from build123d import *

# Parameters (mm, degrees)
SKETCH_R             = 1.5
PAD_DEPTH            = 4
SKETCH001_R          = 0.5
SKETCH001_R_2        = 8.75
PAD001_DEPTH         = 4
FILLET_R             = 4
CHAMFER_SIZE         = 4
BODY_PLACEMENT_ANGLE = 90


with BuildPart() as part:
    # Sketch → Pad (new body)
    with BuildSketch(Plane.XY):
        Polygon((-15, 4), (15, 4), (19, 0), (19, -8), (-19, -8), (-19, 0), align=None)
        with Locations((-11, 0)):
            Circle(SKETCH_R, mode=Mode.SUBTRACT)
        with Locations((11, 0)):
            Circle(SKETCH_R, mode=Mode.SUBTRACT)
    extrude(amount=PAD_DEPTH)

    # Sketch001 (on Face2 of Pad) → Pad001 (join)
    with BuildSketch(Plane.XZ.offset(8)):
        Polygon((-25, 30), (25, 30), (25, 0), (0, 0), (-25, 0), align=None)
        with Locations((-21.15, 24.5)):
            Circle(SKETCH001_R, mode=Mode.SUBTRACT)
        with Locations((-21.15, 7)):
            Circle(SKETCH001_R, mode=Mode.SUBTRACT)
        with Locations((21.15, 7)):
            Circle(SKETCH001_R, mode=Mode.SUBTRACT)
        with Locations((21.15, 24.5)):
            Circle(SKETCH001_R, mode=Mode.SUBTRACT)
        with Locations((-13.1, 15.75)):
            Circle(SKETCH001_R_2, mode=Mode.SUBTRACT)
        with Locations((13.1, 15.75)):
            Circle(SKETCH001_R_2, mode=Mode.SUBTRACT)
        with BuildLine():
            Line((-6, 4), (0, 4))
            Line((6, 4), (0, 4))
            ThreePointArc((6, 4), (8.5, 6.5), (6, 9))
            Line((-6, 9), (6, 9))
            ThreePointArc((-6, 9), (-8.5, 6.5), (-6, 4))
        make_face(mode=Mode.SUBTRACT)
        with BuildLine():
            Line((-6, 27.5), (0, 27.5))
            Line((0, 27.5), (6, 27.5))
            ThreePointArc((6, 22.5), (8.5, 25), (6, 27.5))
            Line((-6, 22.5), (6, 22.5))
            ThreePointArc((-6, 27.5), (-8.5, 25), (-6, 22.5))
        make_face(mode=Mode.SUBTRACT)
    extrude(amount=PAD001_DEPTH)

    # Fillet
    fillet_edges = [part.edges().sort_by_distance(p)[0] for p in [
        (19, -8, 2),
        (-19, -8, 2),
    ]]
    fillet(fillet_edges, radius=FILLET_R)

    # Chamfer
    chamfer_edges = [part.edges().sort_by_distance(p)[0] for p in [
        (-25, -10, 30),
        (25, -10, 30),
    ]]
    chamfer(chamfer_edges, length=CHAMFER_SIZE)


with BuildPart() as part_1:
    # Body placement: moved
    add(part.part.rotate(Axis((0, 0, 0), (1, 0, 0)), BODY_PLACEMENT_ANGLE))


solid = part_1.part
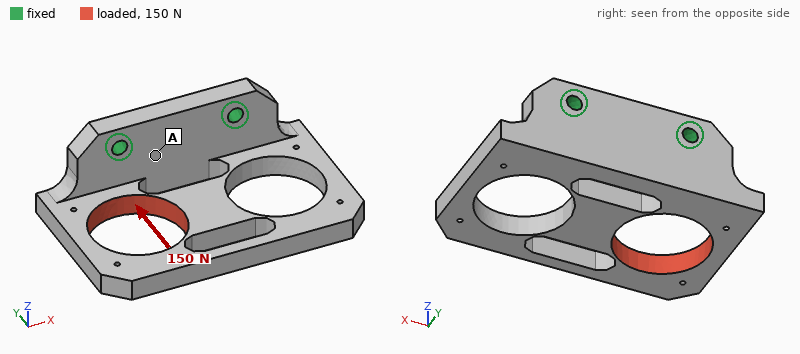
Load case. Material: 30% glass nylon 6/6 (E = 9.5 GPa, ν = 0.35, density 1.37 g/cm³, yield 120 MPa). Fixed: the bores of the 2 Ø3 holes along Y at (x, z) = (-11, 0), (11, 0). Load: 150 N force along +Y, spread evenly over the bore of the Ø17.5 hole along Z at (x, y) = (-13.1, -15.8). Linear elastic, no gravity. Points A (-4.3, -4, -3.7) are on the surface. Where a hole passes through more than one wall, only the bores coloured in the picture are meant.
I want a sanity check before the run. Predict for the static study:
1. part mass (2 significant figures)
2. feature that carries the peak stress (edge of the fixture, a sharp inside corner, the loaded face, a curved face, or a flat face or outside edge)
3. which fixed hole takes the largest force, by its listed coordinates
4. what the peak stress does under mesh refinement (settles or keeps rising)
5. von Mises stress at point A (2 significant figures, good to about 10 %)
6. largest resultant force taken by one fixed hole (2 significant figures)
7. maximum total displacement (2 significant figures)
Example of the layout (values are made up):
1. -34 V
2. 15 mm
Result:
1. 7.0 g
2. edge of the fixture
3. (-11, 0)
4. keeps rising
5. 8.1 MPa
6. 150 N
7. 0.25 mm
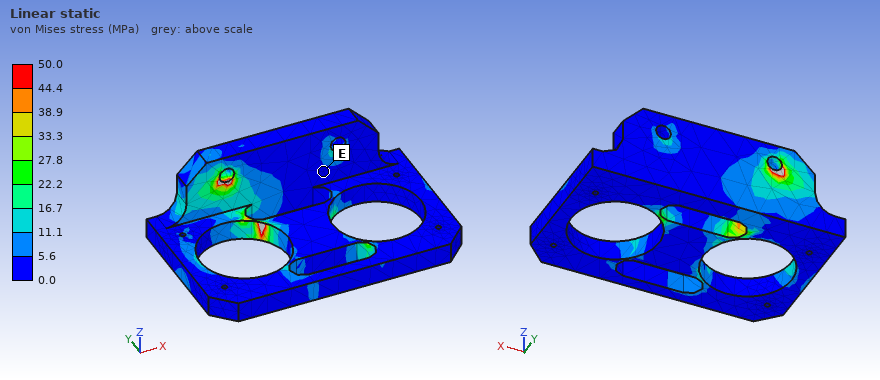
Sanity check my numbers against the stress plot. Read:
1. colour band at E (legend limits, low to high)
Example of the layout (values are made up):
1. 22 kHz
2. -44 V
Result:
1. 0.0 to 5.6 MPa
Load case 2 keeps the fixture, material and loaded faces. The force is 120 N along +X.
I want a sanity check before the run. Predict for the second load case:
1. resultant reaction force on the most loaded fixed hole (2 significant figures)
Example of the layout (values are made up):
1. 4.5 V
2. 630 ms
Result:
1. 95 N
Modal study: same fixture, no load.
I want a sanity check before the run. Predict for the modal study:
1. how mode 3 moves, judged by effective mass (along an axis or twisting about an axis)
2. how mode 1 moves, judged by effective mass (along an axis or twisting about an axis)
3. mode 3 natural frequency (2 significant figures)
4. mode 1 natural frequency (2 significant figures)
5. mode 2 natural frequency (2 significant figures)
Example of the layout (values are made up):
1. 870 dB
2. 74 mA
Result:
1. along X
2. along Z
3. 2900 Hz
4. 1100 Hz
5. 2000 Hz
